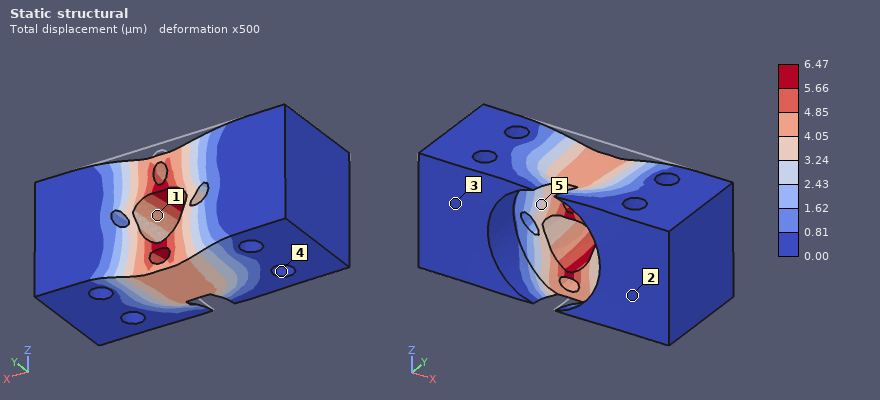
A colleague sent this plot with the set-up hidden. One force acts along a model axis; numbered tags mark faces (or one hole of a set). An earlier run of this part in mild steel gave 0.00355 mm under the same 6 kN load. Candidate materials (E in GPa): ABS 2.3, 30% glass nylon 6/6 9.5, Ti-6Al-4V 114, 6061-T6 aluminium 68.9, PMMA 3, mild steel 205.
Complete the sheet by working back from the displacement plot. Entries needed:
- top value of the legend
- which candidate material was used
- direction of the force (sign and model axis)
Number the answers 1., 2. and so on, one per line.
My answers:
1. 6.47 µm
2. Ti-6Al-4V
3. -Z
